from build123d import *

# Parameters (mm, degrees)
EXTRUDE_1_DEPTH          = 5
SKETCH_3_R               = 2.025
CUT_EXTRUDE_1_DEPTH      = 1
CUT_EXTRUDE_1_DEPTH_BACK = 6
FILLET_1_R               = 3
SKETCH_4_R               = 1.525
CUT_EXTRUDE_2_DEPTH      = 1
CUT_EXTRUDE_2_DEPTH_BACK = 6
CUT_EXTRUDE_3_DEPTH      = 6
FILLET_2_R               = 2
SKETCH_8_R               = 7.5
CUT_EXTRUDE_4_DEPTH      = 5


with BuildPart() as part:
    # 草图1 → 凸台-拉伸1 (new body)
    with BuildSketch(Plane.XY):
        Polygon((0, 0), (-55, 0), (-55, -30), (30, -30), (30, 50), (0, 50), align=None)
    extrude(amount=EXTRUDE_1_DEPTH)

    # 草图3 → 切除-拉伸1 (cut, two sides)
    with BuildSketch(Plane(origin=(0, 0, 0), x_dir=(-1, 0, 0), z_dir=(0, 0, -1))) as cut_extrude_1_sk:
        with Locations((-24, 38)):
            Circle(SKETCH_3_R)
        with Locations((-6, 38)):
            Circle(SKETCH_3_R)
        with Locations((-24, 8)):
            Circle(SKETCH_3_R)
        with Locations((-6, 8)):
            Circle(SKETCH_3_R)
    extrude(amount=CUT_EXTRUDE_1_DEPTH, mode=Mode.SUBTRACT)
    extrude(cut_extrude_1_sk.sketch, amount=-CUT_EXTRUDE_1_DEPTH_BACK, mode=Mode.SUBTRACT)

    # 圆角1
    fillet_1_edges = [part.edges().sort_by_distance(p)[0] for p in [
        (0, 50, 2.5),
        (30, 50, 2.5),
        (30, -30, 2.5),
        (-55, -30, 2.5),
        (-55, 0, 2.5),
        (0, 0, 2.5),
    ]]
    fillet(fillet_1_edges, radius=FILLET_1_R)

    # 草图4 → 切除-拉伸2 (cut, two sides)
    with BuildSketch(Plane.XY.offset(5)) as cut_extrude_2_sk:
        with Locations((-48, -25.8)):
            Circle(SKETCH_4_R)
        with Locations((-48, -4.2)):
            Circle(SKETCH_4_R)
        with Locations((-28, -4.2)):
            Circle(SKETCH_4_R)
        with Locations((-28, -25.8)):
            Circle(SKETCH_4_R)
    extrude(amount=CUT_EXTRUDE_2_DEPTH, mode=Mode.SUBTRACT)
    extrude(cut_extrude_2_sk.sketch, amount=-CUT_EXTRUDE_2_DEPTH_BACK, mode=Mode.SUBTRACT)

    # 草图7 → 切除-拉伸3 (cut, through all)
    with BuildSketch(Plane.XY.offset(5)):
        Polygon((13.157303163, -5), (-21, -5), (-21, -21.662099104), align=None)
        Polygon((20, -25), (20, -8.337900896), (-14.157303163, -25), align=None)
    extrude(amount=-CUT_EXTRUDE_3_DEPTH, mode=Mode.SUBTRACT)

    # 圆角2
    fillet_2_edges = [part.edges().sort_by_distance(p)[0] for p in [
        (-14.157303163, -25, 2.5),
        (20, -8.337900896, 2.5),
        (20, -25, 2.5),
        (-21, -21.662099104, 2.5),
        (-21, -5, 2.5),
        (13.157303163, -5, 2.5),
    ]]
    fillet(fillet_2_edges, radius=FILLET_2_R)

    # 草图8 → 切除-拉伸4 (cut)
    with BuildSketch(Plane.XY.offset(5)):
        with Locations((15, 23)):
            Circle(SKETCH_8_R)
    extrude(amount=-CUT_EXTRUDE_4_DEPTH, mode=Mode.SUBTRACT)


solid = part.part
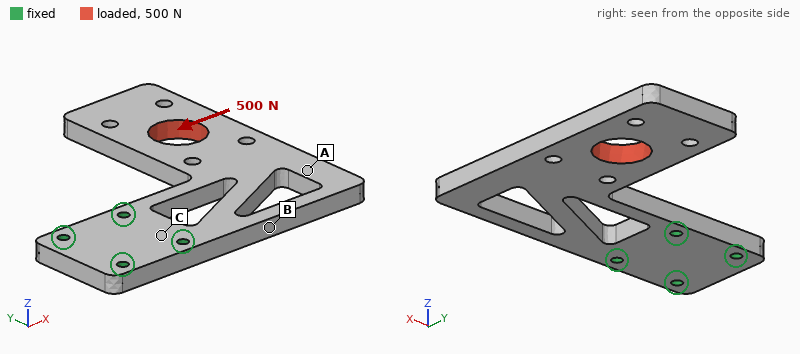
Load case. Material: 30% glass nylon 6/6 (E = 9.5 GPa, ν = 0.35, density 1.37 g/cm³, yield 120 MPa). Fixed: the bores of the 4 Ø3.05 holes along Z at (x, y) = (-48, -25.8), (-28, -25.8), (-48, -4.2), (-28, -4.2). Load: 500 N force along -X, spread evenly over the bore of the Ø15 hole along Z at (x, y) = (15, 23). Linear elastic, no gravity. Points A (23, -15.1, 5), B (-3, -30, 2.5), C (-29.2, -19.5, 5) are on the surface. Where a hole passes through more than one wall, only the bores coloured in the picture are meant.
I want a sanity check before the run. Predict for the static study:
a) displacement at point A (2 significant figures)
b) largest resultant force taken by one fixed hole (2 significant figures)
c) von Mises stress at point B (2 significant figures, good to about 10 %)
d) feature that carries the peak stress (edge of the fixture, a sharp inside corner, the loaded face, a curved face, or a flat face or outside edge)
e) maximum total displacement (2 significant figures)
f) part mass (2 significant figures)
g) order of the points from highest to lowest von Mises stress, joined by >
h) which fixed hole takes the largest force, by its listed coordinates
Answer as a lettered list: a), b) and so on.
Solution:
a) 0.40 mm
b) 1.0 kN
c) 29 MPa
d) a curved face
e) 1.3 mm
f) 22 g
g) B > A > C
h) (-28, -4.2)
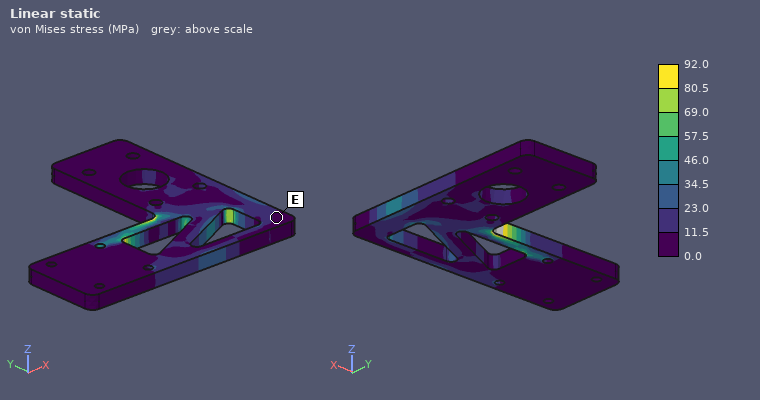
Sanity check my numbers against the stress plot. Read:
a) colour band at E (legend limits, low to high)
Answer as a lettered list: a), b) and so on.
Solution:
a) 0.0 to 11.5 MPa
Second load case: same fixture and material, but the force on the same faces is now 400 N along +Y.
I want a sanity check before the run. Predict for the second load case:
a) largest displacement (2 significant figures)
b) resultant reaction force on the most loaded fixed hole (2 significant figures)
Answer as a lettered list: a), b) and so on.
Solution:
a) 0.53 mm
b) 750 N
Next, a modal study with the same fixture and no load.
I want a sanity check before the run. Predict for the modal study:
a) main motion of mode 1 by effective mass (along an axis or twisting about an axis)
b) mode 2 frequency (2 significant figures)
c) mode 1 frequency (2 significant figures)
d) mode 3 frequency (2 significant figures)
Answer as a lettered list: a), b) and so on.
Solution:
a) along Z
b) 540 Hz
c) 230 Hz
d) 1100 Hz
